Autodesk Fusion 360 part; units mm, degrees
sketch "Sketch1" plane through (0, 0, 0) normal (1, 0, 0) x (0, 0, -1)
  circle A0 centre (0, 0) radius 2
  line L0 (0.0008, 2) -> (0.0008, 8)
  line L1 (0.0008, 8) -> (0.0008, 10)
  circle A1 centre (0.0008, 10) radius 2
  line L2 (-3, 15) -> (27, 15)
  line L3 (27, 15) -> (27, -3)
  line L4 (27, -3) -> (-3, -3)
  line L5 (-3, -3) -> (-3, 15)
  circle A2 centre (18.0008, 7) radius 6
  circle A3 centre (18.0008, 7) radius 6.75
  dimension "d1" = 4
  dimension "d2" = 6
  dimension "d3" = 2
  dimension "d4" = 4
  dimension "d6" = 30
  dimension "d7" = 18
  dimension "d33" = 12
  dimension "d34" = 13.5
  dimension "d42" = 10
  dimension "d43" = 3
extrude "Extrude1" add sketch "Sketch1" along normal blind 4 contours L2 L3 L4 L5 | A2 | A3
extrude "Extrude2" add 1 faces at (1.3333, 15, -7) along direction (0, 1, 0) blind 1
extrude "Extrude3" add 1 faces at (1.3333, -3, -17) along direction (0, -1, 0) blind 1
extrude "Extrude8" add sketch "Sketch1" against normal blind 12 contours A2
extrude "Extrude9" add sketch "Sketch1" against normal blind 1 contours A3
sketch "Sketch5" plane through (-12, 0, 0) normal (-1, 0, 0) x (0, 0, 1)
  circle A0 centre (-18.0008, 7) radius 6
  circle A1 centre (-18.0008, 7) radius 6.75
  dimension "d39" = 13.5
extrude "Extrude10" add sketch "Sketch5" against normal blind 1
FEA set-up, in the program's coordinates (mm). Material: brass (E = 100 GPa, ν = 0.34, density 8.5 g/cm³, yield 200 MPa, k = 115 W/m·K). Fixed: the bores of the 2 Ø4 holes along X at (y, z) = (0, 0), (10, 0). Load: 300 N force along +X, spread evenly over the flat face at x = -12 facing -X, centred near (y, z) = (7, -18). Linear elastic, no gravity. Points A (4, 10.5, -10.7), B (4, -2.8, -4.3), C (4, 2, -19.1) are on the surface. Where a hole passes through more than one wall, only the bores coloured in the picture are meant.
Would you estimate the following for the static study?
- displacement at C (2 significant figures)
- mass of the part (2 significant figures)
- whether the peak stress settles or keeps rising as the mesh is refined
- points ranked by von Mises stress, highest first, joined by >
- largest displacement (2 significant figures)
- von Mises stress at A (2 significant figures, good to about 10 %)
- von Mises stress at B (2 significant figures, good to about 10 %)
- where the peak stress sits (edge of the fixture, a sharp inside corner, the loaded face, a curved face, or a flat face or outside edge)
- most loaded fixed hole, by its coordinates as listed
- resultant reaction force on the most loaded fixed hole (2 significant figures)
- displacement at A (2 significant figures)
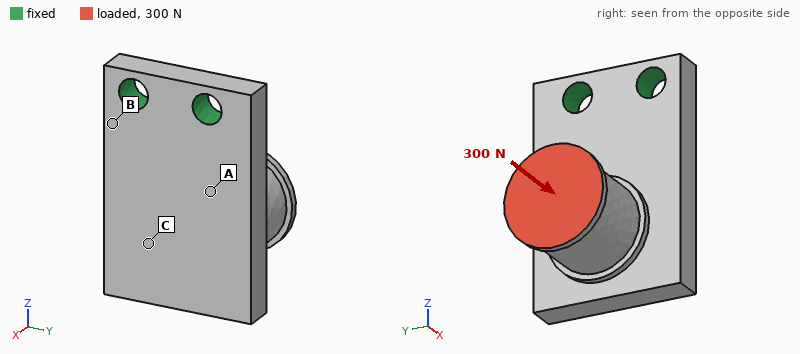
49 µm
32 g
keeps rising
B > A > C
89 µm
37 MPa
68 MPa
edge of the fixture
(10, 0)
200 N
21 µm
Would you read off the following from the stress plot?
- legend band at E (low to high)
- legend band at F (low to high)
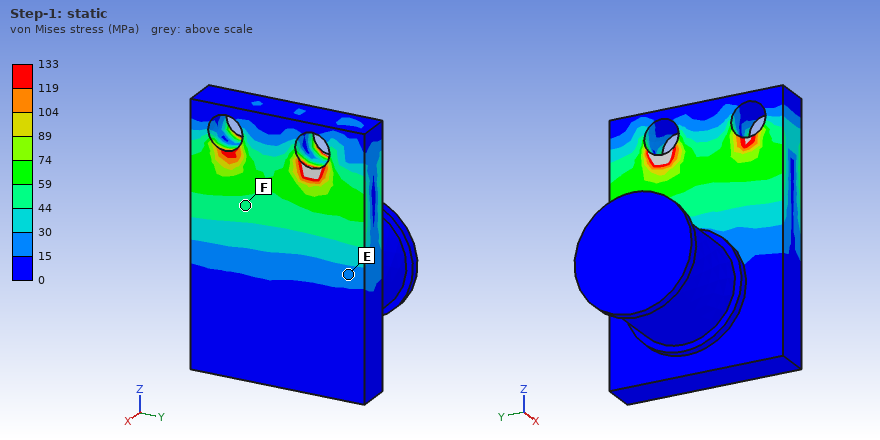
15 to 30 MPa
44 to 59 MPa
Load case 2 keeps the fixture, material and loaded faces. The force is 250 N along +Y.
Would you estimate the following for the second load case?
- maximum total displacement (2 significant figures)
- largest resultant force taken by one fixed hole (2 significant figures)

38 µm
430 N
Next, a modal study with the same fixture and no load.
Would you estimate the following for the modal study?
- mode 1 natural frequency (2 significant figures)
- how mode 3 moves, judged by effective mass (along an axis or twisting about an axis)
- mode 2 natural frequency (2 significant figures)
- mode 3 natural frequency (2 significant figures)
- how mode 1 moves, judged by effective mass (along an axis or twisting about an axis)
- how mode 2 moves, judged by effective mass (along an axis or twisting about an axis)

2200 Hz
along Y
5200 Hz
9600 Hz
along X
along Y
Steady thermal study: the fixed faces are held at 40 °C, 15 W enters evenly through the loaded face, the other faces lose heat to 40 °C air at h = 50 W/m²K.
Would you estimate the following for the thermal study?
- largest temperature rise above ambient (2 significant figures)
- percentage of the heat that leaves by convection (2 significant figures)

37 K
11 %
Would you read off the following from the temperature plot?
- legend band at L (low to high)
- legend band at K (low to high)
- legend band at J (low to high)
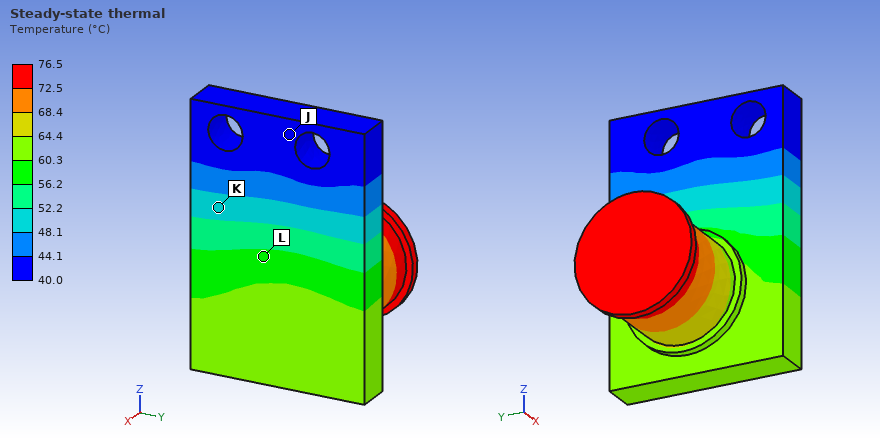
56.2 to 60.3 °C
48.1 to 52.2 °C
40.0 to 44.1 °C
